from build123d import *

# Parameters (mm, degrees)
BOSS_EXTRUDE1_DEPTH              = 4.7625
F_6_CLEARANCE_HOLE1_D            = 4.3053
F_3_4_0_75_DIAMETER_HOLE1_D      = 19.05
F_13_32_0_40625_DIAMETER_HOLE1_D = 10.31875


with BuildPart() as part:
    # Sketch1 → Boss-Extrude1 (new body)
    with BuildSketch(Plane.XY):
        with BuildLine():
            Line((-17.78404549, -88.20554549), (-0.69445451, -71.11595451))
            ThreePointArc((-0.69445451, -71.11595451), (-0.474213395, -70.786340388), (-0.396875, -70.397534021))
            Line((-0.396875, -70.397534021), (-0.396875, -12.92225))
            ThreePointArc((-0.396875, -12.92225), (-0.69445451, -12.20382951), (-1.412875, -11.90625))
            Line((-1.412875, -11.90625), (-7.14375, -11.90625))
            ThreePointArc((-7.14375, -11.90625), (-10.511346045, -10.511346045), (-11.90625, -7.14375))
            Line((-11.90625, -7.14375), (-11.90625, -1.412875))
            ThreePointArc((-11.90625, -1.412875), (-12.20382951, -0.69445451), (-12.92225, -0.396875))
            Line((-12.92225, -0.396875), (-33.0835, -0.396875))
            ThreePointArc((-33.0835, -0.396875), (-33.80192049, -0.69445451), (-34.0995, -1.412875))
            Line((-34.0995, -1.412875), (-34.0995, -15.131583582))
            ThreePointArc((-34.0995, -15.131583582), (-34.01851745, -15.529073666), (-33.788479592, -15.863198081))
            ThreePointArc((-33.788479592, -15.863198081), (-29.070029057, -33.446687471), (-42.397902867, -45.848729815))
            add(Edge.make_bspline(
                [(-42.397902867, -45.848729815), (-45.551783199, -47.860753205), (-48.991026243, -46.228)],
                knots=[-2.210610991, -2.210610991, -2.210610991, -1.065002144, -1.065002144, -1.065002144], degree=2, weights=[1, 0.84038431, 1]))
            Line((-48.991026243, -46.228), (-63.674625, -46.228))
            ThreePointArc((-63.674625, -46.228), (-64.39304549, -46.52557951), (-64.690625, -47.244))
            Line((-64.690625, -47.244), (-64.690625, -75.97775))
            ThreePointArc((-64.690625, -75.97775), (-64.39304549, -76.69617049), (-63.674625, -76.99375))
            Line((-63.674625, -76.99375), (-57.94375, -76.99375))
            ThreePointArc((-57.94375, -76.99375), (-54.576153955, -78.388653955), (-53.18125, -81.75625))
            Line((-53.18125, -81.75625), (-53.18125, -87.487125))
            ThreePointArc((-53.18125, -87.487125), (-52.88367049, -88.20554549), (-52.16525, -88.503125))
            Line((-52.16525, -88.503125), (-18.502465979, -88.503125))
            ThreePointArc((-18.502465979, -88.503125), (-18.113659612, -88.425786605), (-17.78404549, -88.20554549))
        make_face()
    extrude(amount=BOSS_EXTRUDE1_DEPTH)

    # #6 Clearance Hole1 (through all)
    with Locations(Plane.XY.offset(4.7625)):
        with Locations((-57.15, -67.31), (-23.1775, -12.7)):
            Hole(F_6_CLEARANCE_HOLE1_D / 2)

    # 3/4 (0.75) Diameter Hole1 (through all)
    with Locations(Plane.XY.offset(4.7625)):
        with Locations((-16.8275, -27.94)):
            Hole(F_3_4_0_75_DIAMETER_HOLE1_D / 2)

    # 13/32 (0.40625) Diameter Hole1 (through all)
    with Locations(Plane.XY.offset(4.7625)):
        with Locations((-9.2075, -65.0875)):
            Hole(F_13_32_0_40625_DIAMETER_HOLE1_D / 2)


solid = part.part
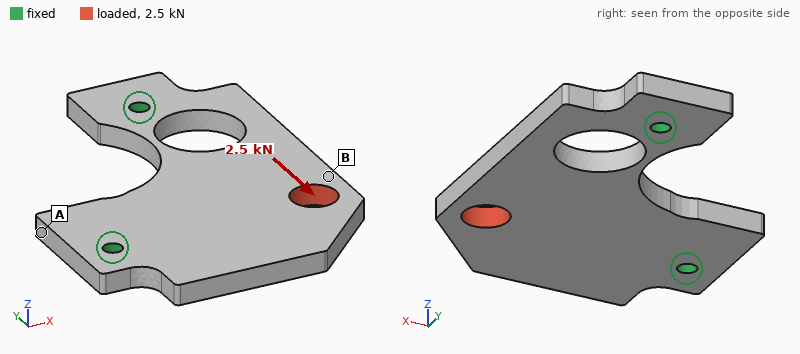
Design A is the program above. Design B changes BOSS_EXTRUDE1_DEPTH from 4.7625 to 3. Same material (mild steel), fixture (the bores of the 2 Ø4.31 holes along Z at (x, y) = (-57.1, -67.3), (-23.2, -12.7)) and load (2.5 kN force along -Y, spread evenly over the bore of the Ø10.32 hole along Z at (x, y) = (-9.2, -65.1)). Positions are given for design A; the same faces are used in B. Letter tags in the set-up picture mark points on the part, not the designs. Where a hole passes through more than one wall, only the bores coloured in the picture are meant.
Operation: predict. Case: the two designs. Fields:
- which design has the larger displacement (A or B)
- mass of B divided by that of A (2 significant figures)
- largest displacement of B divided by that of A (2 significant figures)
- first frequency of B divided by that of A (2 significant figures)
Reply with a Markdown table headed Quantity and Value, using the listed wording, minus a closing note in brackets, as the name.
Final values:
| Quantity | Value |
|---|---|
| which design has the larger displacement | B |
| mass of B divided by that of A | 0.63 |
| largest displacement of B divided by that of A | 1.6 |
| first frequency of B divided by that of A | 0.66 |
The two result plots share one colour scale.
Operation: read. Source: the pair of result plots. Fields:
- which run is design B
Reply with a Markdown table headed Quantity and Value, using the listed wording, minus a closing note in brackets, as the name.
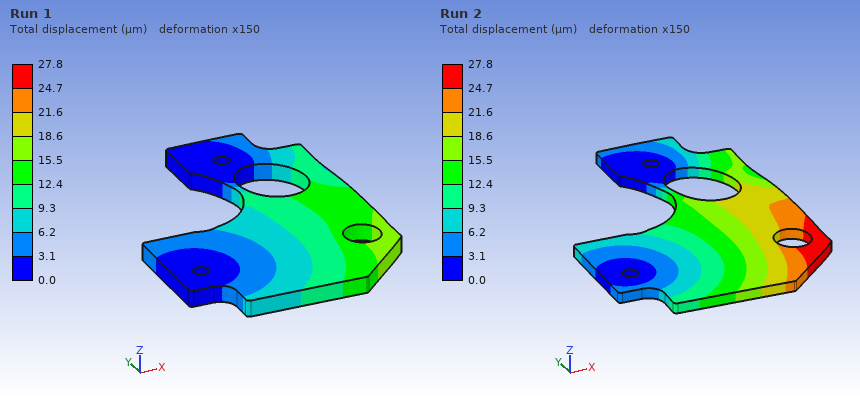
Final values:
| Quantity | Value |
|---|---|
| which run is design B | Run 2 |
